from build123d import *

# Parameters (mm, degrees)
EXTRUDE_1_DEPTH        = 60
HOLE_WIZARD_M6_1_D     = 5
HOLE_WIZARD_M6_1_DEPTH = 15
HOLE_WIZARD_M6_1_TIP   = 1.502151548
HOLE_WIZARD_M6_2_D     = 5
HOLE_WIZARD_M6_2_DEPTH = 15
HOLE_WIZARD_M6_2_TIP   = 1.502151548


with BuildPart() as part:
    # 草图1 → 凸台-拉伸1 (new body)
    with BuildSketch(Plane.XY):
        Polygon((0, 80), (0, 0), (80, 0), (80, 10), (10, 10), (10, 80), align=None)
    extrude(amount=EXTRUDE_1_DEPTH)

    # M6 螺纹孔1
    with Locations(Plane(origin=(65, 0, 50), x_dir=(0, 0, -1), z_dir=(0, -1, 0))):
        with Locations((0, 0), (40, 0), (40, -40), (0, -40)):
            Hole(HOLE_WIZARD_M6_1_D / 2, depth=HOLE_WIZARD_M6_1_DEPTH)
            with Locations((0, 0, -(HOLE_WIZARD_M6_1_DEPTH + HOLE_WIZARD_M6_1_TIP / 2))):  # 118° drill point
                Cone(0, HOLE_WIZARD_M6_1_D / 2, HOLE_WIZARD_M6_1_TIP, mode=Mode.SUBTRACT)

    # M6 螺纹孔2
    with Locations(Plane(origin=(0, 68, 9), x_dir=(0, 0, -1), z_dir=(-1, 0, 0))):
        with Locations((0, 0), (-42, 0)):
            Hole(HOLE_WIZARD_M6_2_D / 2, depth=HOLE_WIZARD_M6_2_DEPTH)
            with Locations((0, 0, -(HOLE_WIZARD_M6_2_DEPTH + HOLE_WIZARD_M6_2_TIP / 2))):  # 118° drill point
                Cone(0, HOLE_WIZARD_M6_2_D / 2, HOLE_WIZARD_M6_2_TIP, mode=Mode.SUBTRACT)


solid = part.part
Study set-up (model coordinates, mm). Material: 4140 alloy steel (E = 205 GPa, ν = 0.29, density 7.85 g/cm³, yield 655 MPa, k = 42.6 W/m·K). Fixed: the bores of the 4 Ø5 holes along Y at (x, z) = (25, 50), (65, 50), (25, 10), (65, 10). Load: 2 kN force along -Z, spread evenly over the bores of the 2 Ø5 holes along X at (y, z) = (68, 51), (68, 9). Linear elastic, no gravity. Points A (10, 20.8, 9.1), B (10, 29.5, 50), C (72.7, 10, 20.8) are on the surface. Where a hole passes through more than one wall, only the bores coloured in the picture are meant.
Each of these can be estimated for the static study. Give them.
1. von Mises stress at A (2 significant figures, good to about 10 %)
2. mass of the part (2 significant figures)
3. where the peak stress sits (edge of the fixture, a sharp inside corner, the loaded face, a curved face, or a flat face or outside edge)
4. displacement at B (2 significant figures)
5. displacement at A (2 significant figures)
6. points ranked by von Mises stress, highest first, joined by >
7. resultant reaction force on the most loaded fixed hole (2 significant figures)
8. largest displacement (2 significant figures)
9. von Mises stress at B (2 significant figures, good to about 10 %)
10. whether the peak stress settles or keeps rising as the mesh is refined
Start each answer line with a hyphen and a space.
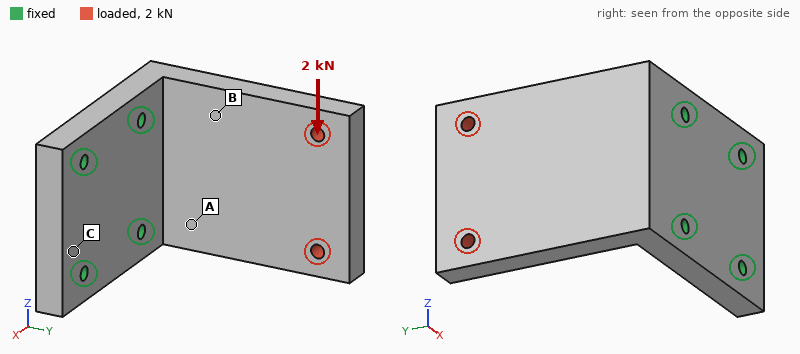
- 31 MPa
- 700 g
- edge of the fixture
- 21 µm
- 16 µm
- A > B > C
- 3.2 kN
- 54 µm
- 20 MPa
- keeps rising
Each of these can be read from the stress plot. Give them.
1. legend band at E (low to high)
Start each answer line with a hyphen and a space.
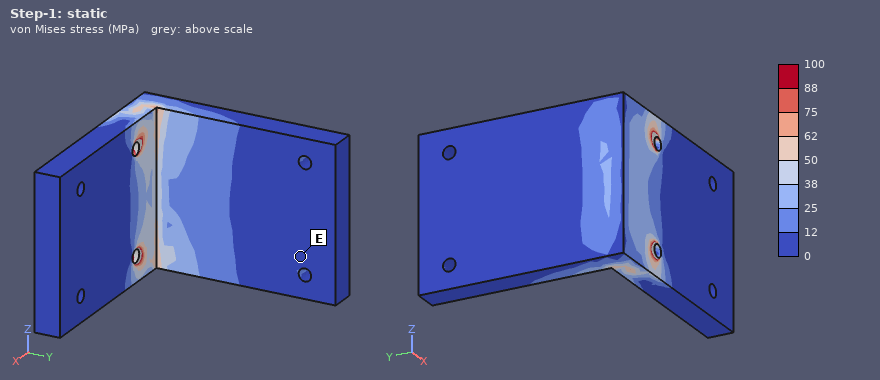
- 0 to 12 MPa
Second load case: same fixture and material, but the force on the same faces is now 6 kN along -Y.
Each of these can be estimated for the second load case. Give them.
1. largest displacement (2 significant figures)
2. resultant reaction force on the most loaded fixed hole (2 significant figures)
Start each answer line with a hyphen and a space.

- 0.11 mm
- 3.4 kN
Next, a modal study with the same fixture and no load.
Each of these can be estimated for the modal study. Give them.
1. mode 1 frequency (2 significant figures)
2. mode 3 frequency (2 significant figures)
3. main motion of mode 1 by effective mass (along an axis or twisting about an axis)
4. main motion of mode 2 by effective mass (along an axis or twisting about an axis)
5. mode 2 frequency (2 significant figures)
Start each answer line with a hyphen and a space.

- 1100 Hz
- 4000 Hz
- along X
- along Z
- 2500 Hz
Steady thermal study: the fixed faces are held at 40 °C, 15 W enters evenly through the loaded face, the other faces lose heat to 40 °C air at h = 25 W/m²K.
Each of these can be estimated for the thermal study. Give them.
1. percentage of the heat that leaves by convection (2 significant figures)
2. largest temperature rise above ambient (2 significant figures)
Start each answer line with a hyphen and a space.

- 42 %
- 37 K
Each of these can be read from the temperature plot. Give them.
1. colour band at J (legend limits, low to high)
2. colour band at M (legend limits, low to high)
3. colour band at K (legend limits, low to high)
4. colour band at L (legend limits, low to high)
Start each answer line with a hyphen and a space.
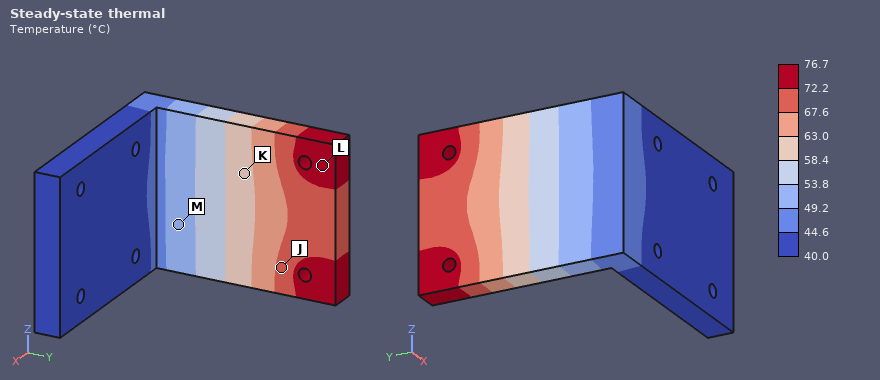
- 67.6 to 72.2 °C
- 49.2 to 53.8 °C
- 58.4 to 63.0 °C
- 72.2 to 76.7 °C
